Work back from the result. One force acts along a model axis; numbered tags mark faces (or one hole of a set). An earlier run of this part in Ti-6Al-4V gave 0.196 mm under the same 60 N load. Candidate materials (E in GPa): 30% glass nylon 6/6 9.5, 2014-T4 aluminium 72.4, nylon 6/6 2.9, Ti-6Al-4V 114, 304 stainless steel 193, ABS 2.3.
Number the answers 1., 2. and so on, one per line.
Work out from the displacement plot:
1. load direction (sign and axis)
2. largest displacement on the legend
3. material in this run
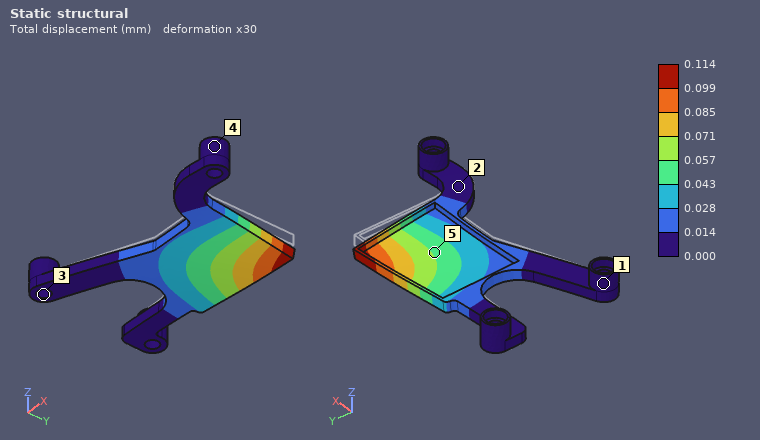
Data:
1. -Z
2. 0.114 mm
3. 304 stainless steel
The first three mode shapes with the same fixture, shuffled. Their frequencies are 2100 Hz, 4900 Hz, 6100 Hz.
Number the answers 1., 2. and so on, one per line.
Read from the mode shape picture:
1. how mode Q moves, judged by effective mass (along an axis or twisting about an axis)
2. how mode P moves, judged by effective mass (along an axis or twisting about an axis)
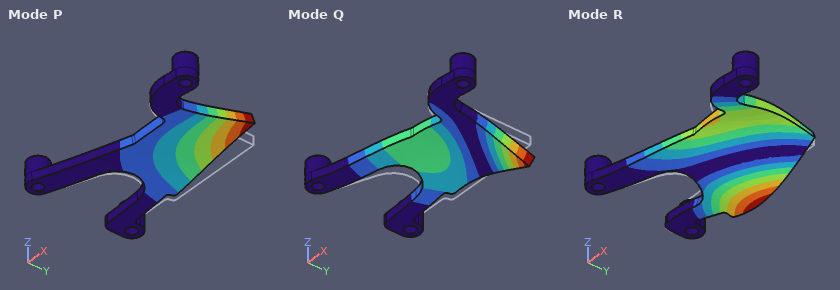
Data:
1. along Z
2. along Z
